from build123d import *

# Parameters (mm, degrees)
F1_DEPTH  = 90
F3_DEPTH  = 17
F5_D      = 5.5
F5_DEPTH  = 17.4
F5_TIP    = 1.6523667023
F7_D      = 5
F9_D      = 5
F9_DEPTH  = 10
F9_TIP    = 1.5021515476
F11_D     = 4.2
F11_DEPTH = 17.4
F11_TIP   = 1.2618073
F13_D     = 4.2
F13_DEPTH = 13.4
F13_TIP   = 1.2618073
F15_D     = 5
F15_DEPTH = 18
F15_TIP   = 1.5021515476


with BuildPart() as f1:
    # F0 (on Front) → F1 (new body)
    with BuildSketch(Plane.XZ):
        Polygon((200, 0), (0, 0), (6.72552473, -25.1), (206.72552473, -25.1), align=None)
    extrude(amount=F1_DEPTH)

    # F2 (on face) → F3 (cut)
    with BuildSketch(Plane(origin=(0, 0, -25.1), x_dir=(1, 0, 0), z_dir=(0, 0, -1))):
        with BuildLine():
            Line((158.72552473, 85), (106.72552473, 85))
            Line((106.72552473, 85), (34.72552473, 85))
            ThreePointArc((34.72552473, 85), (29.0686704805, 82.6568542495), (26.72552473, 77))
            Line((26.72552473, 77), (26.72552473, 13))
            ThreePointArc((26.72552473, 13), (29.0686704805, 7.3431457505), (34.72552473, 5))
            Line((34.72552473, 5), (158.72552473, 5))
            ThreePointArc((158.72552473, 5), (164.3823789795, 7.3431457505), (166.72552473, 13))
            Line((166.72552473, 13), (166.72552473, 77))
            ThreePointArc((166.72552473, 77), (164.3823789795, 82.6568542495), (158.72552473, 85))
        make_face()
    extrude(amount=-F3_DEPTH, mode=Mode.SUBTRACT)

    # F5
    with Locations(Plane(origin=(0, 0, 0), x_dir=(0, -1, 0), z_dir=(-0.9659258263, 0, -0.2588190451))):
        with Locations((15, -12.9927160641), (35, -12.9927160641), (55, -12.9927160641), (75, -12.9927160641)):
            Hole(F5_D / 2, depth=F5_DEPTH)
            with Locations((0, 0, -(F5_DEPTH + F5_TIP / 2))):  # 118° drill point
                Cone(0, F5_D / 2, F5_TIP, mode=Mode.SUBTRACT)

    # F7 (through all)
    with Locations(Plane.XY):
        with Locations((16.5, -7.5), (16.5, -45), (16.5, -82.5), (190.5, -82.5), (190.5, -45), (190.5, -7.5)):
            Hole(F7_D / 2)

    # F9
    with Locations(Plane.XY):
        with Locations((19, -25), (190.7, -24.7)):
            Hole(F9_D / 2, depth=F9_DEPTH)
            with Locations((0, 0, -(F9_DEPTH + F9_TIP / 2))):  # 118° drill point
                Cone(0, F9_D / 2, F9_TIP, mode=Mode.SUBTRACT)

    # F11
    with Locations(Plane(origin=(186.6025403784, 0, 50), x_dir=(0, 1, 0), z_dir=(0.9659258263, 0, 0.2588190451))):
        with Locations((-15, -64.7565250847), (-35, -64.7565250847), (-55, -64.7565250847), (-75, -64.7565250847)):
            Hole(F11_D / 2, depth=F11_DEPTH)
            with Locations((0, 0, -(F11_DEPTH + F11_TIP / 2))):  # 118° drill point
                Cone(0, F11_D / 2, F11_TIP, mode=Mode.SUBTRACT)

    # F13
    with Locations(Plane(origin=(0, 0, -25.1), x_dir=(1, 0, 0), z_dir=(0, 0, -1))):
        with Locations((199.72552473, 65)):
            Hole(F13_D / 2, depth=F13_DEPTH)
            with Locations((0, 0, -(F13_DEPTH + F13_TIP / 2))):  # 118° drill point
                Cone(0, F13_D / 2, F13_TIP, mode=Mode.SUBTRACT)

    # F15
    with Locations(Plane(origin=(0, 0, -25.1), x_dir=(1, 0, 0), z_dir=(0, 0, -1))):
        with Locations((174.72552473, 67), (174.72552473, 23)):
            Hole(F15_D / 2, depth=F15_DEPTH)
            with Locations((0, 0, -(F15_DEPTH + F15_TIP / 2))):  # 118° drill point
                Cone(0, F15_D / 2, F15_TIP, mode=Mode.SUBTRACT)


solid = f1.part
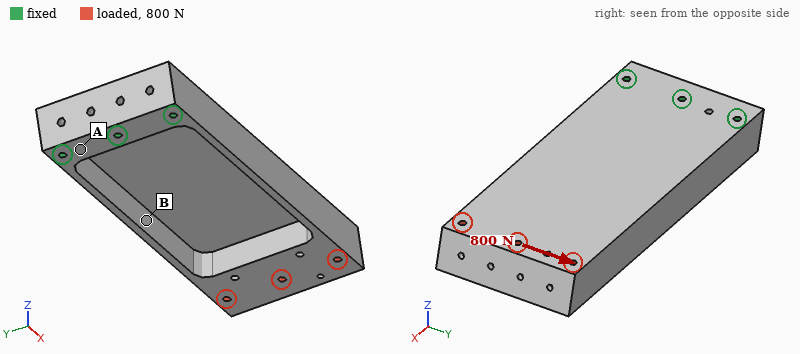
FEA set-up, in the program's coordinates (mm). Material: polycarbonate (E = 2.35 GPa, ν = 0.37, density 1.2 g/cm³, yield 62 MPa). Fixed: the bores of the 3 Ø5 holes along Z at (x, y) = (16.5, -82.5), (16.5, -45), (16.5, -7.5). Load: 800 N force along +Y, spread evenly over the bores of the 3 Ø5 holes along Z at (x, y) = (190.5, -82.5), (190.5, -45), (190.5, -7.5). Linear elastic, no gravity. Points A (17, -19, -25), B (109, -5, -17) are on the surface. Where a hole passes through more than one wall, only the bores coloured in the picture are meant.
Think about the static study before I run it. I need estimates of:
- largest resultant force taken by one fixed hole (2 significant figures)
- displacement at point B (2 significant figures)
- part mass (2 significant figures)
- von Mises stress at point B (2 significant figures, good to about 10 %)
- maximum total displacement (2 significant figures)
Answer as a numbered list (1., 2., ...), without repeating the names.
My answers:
1. 1.8 kN
2. 1.0 mm
3. 310 g
4. 4.1 MPa
5. 2.5 mm
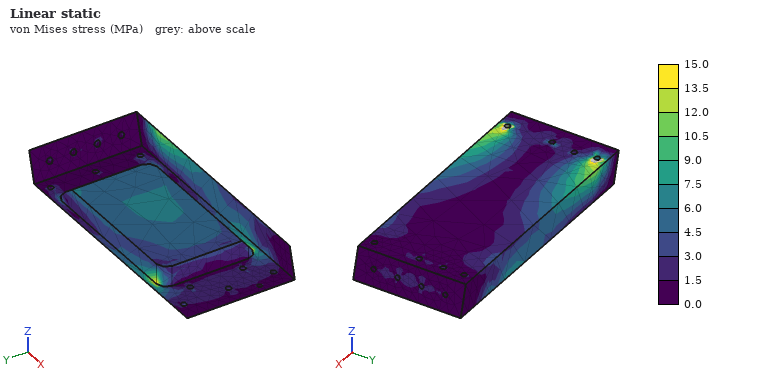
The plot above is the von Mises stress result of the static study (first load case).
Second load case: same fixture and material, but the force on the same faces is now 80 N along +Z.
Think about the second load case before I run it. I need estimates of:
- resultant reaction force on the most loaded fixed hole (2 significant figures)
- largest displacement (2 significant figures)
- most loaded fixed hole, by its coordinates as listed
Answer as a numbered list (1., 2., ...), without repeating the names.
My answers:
1. 290 N
2. 2.3 mm
3. (16.5, -45)
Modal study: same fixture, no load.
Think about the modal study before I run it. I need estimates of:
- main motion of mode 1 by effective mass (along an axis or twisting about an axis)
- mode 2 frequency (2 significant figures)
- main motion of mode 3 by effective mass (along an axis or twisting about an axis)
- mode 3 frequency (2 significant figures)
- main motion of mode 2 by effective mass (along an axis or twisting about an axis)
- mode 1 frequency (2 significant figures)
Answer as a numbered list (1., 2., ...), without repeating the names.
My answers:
1. along Z
2. 240 Hz
3. along Y
4. 460 Hz
5. along Y
6. 95 Hz
